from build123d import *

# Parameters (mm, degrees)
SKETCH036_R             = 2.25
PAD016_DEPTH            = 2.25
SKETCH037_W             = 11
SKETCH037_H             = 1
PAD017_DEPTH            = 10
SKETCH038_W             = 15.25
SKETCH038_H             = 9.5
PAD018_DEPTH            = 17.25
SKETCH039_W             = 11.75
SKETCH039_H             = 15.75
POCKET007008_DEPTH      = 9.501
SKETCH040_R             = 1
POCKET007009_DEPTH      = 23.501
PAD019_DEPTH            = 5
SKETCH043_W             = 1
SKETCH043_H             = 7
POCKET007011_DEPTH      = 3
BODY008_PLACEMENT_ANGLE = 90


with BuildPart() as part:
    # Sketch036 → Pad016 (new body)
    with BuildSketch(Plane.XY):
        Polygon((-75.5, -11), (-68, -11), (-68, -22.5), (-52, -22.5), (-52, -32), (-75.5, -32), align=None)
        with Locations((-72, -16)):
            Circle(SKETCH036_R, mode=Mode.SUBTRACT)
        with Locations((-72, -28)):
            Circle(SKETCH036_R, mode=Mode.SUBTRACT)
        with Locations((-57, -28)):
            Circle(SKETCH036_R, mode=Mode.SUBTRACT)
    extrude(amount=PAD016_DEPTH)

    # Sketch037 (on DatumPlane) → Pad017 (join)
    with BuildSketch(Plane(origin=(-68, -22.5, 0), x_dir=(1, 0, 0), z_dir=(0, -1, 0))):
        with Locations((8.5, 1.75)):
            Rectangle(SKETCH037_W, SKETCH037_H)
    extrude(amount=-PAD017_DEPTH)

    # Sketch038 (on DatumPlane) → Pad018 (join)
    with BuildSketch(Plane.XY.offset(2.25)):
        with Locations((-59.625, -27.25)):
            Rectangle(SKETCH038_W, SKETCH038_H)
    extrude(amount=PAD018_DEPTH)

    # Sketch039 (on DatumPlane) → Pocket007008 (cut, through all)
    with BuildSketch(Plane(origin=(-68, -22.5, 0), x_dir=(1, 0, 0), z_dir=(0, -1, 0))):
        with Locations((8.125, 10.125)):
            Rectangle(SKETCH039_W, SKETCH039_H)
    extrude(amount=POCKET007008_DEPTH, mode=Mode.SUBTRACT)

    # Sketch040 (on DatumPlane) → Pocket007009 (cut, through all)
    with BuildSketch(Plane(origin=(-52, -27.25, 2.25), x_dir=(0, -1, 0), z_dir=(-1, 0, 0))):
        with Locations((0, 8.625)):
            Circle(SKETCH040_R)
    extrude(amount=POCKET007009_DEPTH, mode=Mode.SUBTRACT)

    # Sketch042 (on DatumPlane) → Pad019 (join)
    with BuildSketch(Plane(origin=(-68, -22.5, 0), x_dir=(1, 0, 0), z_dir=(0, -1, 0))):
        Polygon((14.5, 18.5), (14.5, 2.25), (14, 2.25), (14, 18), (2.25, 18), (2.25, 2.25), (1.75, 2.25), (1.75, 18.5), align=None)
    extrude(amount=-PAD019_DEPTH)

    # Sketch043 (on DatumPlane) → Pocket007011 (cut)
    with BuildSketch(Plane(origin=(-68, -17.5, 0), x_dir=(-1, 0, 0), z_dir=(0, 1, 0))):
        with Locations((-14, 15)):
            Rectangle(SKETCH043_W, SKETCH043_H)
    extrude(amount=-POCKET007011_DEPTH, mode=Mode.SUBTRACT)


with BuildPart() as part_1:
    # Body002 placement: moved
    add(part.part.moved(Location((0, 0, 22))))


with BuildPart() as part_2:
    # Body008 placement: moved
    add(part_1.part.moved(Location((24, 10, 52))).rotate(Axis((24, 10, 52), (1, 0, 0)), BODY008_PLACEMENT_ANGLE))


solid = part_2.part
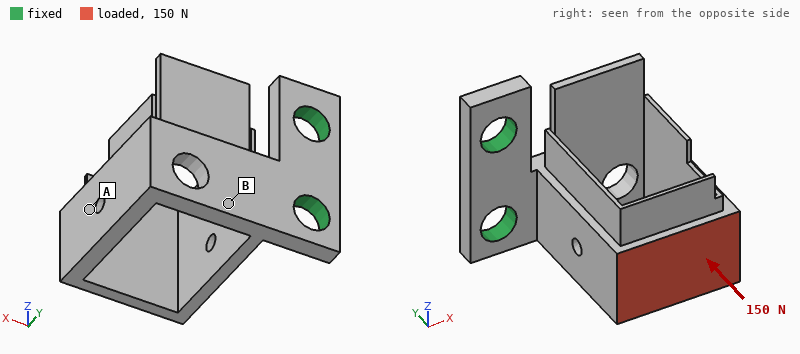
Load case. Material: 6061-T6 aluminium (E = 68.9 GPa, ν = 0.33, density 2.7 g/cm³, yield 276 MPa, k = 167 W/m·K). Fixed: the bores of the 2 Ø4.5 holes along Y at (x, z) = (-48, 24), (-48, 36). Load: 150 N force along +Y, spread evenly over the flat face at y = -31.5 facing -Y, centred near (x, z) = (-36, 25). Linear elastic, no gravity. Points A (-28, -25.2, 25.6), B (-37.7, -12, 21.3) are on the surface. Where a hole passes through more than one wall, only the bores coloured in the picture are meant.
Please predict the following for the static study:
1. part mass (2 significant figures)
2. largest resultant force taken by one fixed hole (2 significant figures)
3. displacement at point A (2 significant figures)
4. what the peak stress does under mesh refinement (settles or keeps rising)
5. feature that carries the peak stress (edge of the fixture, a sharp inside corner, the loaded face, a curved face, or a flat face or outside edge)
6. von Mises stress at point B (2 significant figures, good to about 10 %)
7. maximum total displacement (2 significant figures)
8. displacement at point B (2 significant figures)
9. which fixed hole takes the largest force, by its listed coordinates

4.1 g
150 N
0.25 mm
keeps rising
edge of the fixture
59 MPa
0.30 mm
0.065 mm
(-48, 24)
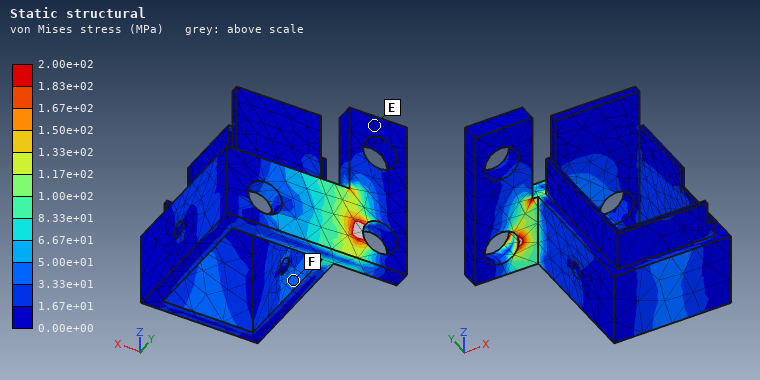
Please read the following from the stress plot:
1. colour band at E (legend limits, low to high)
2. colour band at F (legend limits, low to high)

0.00e+00 to 1.67e+01 MPa
3.33e+01 to 5.00e+01 MPa
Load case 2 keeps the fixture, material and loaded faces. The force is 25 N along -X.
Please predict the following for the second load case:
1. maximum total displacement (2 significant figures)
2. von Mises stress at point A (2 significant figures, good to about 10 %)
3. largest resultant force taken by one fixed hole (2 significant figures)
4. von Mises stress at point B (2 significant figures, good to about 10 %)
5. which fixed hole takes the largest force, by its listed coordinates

0.13 mm
5.3 MPa
24 N
20 MPa
(-48, 24)
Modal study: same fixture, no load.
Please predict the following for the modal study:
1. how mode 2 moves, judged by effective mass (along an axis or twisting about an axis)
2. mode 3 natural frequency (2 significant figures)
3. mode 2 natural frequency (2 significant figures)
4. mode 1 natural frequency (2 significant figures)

along Z
6100 Hz
3500 Hz
1800 Hz
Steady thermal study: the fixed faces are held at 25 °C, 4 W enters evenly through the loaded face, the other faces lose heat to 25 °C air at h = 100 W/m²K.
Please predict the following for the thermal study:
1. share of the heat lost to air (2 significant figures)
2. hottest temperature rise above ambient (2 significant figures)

40 %
16 K
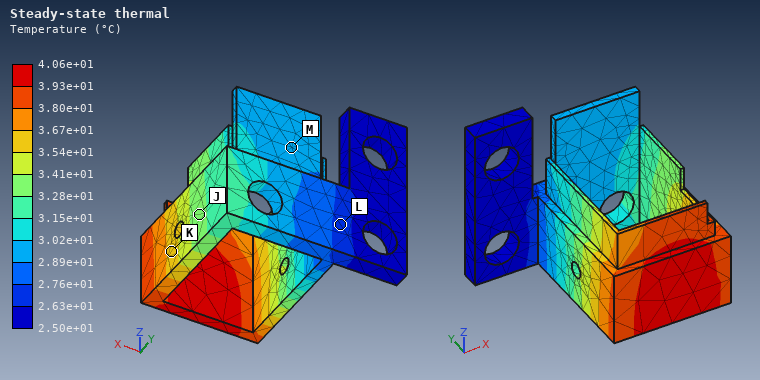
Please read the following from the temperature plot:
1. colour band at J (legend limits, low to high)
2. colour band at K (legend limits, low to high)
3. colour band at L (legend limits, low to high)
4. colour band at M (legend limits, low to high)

3.28e+01 to 3.41e+01 °C
3.54e+01 to 3.67e+01 °C
2.63e+01 to 2.76e+01 °C
2.89e+01 to 3.02e+01 °C
